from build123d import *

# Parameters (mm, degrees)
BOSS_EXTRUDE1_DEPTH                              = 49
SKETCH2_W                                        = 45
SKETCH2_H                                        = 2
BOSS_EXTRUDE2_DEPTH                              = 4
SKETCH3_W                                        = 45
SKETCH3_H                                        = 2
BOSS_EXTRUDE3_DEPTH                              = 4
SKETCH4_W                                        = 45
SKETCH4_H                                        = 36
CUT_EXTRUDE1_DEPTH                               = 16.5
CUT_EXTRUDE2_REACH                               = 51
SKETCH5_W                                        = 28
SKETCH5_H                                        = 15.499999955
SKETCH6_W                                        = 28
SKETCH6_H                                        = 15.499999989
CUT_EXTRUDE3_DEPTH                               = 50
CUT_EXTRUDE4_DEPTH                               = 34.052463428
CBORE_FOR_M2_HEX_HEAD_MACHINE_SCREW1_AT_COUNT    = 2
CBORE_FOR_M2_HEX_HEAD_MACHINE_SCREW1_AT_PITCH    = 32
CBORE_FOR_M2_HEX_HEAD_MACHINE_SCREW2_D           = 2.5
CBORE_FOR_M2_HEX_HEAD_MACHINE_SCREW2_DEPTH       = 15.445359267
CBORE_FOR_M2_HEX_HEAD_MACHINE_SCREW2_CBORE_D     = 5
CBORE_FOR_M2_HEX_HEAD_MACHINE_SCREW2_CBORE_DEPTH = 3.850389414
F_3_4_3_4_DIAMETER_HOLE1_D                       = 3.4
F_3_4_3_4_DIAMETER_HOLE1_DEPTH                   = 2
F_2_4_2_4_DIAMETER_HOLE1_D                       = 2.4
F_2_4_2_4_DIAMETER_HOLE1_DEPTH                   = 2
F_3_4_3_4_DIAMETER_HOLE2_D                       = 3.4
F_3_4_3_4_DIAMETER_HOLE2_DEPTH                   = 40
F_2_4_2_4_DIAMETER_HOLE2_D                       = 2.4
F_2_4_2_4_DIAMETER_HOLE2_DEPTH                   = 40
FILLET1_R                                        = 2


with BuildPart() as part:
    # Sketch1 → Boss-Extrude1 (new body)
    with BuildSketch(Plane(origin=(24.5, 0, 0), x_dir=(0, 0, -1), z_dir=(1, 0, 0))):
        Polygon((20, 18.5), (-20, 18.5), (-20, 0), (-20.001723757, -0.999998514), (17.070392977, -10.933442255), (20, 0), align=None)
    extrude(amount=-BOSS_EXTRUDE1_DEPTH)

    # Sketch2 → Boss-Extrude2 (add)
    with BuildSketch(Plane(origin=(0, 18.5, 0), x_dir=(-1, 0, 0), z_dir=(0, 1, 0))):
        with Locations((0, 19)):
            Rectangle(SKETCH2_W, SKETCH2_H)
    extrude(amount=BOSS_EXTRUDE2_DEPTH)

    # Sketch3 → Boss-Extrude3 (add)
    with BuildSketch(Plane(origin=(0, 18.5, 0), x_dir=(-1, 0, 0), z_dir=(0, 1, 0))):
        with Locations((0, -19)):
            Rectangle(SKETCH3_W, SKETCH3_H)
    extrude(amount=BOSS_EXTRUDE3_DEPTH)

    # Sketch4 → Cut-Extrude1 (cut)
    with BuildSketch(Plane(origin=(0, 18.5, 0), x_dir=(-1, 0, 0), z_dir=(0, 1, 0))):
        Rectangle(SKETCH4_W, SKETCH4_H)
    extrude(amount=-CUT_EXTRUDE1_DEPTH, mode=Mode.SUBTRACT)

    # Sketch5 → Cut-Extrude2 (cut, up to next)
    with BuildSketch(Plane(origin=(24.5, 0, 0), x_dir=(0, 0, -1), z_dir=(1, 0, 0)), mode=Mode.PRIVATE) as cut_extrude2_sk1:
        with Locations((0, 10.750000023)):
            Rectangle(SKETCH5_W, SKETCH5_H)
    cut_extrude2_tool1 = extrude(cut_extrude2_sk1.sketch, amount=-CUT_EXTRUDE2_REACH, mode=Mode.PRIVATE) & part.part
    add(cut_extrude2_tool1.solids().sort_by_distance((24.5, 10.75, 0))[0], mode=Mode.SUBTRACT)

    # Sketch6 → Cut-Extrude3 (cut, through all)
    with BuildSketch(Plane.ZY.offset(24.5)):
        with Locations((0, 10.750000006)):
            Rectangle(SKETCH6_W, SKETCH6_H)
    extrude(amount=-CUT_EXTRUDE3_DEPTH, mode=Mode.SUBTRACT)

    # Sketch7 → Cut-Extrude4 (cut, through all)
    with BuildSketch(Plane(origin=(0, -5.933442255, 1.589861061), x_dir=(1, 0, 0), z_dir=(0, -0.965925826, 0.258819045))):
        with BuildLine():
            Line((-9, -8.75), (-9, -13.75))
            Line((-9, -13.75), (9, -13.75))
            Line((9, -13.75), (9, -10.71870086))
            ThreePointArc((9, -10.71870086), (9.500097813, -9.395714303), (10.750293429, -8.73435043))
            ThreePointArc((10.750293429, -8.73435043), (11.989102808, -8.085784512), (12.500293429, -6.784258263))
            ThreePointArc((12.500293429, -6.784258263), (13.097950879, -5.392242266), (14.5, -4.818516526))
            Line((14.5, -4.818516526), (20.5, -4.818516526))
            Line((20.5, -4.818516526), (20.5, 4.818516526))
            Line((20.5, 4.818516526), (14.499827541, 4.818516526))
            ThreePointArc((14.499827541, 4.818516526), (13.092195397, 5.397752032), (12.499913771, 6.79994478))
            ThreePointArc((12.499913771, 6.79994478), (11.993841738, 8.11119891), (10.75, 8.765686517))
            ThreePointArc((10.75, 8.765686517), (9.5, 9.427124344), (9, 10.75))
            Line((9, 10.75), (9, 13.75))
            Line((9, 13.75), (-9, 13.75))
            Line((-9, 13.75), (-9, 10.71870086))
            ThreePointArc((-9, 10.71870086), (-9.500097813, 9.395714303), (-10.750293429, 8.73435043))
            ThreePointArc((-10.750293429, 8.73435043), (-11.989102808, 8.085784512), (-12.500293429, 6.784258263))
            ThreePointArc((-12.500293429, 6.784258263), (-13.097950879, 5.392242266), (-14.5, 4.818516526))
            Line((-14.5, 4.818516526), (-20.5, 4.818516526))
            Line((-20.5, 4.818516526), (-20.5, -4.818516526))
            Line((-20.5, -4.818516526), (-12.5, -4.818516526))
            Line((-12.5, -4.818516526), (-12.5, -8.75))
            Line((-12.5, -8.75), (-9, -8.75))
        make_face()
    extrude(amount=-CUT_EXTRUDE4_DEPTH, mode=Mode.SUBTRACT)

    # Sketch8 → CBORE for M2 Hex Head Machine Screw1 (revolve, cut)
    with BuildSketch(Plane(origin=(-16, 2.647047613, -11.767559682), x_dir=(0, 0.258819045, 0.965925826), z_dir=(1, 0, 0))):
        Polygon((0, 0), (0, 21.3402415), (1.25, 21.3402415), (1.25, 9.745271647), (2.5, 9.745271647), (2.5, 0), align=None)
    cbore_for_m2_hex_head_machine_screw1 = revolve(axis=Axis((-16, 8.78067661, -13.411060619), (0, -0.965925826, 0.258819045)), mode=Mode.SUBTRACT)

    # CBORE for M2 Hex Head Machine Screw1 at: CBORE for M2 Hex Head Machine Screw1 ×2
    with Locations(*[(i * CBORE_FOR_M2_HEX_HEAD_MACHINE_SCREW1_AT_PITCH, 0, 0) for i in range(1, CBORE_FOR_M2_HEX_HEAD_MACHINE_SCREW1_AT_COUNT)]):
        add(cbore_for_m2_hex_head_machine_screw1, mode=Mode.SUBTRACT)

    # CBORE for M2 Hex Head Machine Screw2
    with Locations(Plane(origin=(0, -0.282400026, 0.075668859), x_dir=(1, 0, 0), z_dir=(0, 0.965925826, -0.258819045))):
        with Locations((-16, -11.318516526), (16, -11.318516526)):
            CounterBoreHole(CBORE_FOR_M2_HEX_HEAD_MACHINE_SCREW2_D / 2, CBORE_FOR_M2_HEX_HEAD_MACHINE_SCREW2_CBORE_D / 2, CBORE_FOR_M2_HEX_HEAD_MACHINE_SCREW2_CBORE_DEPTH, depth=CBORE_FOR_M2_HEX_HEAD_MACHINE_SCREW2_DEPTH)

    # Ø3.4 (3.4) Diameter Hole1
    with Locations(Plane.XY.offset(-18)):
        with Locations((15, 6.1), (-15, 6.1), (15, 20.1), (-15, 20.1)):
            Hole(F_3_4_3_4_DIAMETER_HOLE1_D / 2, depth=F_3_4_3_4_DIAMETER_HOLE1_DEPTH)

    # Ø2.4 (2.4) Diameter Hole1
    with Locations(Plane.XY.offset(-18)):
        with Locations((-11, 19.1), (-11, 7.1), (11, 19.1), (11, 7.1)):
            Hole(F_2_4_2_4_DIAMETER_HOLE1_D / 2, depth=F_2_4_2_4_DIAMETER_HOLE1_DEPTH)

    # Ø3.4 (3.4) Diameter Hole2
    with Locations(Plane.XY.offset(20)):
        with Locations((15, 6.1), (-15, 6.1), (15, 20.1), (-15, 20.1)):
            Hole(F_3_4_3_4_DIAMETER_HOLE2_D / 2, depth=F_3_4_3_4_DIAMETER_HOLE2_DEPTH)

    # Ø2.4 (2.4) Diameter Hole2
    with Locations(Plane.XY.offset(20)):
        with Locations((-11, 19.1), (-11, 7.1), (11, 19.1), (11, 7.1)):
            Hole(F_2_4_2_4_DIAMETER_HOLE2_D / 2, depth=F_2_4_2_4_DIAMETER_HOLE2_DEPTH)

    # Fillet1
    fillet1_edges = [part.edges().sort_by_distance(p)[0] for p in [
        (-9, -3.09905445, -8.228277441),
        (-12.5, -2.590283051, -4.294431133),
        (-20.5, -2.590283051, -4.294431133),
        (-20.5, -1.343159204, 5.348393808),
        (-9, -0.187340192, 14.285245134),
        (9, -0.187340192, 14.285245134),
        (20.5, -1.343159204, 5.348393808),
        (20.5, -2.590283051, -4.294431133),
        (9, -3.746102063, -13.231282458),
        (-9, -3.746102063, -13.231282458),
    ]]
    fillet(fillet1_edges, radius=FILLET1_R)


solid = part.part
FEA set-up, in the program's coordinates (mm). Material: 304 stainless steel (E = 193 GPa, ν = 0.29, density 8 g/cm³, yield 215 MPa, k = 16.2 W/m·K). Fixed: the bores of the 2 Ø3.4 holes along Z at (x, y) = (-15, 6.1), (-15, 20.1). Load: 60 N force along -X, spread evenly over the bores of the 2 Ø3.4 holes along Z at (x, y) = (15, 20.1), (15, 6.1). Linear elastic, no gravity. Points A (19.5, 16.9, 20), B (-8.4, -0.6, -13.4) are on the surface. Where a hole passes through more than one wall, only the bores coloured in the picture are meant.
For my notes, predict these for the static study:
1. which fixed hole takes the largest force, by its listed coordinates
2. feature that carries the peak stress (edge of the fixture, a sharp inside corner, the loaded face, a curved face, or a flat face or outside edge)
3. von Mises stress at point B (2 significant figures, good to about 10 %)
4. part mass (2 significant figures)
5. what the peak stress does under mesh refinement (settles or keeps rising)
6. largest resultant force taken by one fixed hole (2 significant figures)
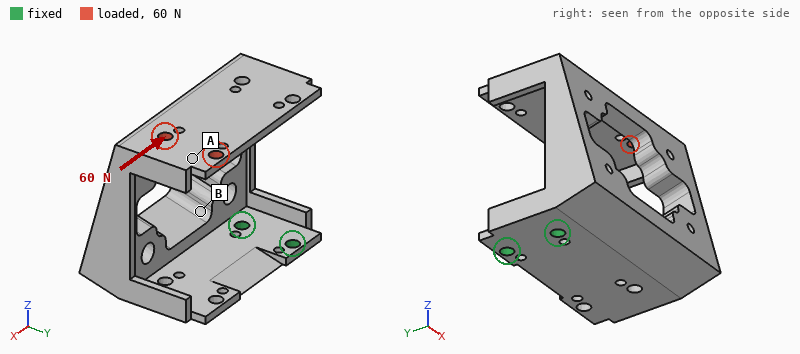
(-15, 20.1)
edge of the fixture
16 MPa
100 g
keeps rising
40 N
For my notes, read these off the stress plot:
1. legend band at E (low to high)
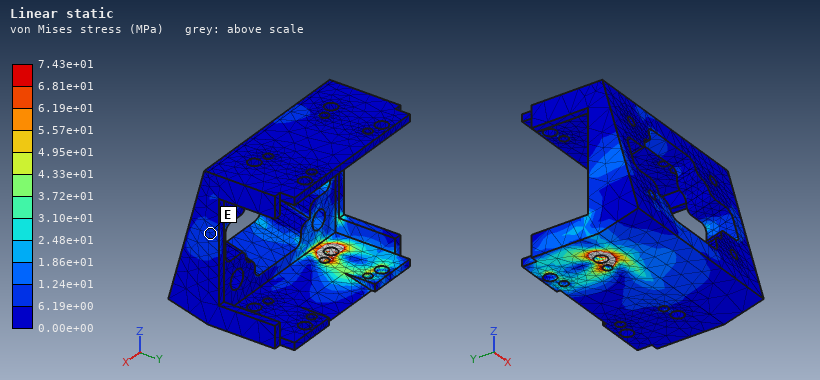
6.19e+00 to 1.24e+01 MPa
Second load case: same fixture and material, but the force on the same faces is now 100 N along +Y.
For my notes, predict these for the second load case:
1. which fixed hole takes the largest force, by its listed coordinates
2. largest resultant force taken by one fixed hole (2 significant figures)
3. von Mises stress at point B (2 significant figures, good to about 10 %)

(-15, 20.1)
280 N
16 MPa
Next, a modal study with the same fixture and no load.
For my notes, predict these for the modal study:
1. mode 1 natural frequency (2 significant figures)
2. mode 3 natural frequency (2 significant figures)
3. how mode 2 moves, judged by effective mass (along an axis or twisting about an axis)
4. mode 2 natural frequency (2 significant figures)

580 Hz
2400 Hz
along Y
730 Hz
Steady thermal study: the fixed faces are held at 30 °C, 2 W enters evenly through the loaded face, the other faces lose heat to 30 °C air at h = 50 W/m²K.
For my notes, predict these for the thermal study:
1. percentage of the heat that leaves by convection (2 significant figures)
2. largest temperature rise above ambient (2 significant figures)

98 %
35 K
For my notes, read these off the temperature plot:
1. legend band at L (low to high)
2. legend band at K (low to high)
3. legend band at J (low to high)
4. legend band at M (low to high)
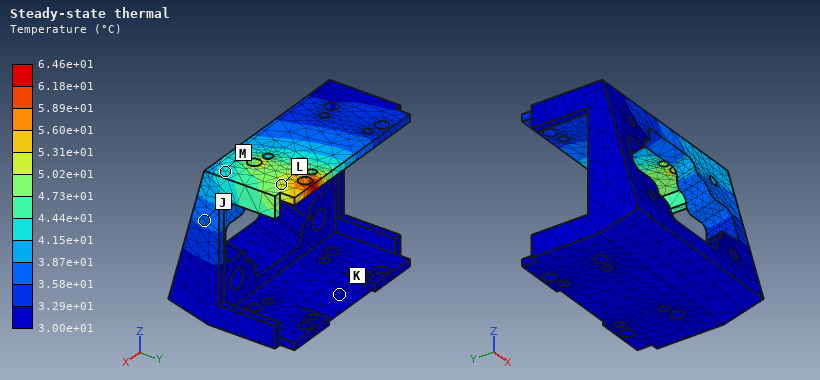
5.02e+01 to 5.31e+01 °C
3.00e+01 to 3.29e+01 °C
3.58e+01 to 3.87e+01 °C
4.15e+01 to 4.44e+01 °C
